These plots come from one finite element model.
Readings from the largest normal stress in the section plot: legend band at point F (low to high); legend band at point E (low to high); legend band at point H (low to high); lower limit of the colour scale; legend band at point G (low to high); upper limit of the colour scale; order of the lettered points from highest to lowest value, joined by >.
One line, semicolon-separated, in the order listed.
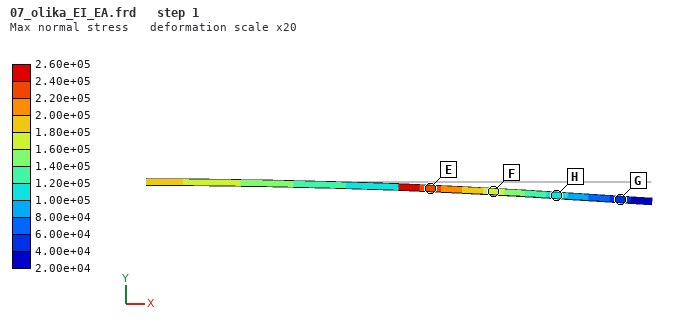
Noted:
1.60e+05 to 1.80e+05; 2.20e+05 to 2.40e+05; 1.00e+05 to 1.20e+05; 2.00e+04; 4.00e+04 to 6.00e+04; 2.60e+05; E > F > H > G
